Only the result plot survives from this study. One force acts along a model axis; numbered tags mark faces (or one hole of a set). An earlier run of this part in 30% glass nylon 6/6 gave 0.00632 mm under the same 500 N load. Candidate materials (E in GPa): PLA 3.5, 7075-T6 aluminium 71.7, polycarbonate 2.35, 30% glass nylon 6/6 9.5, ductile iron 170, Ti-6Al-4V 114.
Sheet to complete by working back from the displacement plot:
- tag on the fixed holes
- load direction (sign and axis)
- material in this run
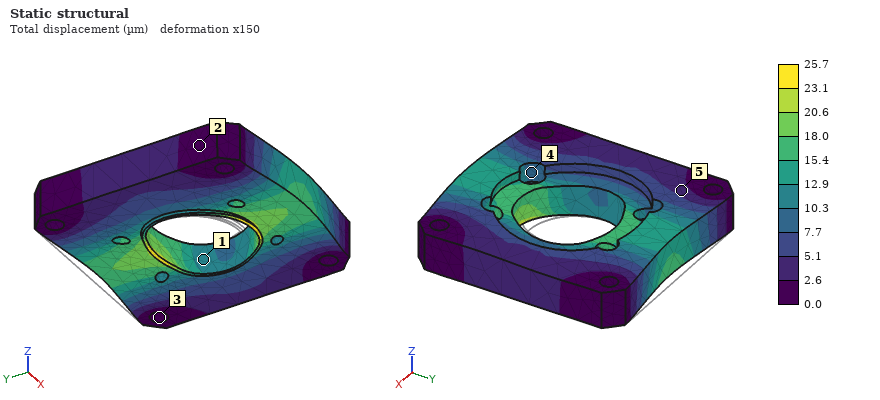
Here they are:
3
-Y
polycarbonate
